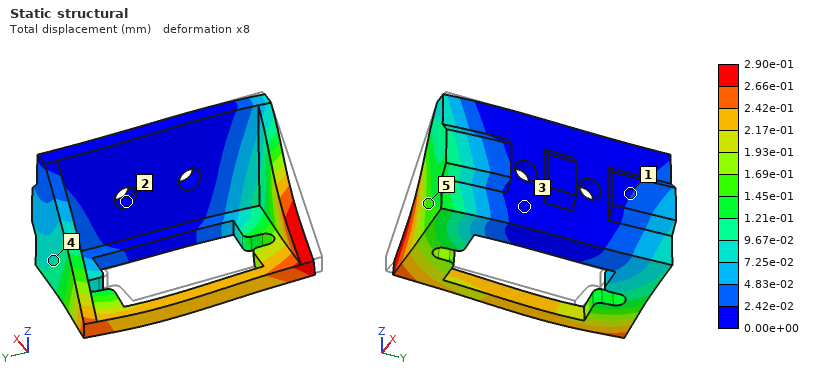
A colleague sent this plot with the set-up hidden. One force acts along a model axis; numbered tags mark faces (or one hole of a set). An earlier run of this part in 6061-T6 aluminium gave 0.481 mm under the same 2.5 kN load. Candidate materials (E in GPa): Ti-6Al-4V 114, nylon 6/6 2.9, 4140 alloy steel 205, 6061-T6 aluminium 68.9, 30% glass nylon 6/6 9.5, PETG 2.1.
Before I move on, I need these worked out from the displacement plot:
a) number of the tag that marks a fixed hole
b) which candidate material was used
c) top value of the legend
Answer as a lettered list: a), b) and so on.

a) 2
b) Ti-6Al-4V
c) 2.90e-01 mm
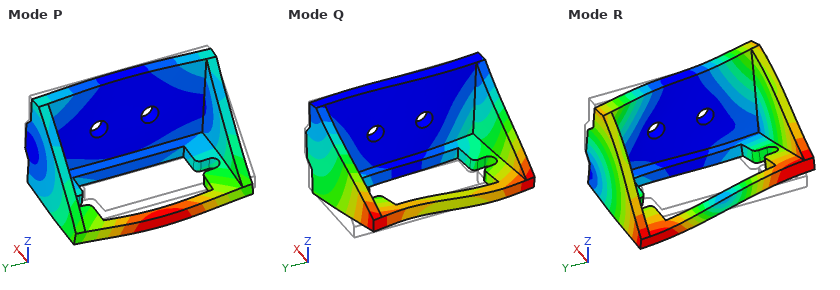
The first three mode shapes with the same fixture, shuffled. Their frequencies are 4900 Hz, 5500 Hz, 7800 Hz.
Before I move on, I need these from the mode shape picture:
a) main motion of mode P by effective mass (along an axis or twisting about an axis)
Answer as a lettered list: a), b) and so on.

a) along Z
